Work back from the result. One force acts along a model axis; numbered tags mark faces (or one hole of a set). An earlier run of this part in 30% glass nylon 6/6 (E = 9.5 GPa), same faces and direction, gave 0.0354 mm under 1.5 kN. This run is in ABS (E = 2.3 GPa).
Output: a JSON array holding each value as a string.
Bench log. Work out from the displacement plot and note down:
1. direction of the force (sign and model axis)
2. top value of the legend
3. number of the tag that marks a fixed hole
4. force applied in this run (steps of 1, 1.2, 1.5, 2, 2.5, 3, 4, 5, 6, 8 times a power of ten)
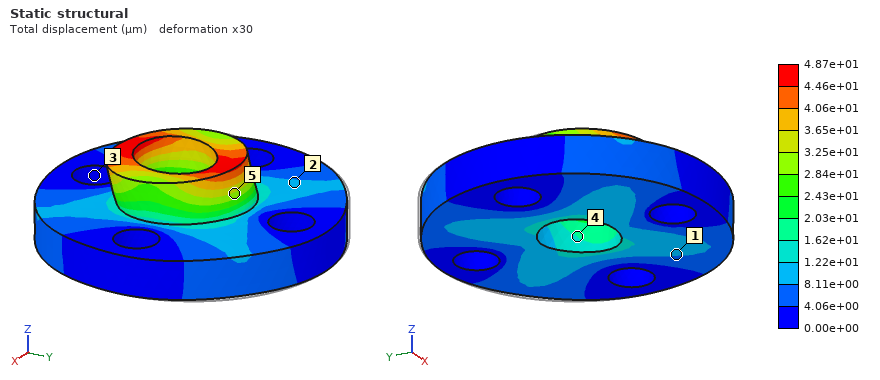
["-Y", "4.87e+01 µm", "3", "500 N"]
